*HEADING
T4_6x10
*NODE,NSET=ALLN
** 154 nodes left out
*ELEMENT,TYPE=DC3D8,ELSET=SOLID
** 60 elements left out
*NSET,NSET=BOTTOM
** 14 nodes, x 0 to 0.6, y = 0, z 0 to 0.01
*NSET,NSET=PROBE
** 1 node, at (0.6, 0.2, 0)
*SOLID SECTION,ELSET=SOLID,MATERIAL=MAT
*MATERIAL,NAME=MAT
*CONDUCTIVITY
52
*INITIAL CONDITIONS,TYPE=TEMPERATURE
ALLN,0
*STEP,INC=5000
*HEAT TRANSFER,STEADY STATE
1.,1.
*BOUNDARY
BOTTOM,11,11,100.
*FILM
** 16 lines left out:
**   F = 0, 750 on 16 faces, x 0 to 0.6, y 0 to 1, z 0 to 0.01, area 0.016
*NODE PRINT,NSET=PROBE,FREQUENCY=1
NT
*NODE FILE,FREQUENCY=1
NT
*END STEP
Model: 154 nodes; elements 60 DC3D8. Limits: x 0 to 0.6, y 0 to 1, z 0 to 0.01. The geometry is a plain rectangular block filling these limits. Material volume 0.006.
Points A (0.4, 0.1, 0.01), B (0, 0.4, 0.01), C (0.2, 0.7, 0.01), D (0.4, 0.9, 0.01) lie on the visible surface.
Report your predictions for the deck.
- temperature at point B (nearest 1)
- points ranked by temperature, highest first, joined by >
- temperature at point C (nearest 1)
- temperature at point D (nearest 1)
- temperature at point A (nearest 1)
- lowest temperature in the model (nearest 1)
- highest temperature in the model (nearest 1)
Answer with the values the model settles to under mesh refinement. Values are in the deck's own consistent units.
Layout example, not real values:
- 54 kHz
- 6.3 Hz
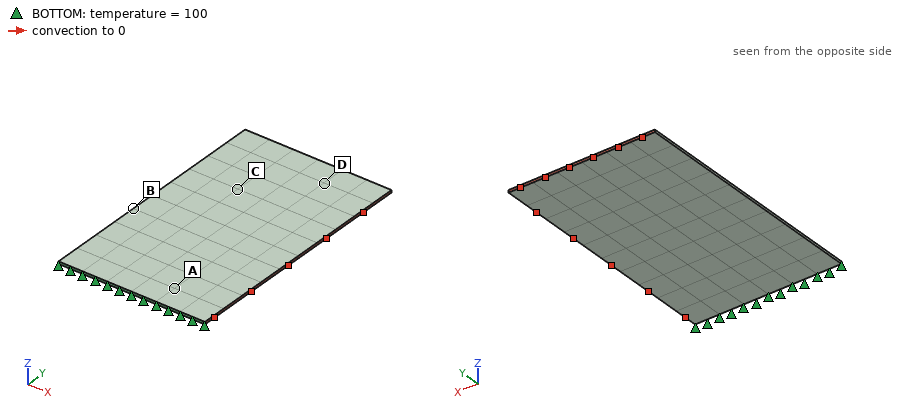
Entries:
- 45
- A > B > C > D
- 18
- 5
- 75
- 1
- 100
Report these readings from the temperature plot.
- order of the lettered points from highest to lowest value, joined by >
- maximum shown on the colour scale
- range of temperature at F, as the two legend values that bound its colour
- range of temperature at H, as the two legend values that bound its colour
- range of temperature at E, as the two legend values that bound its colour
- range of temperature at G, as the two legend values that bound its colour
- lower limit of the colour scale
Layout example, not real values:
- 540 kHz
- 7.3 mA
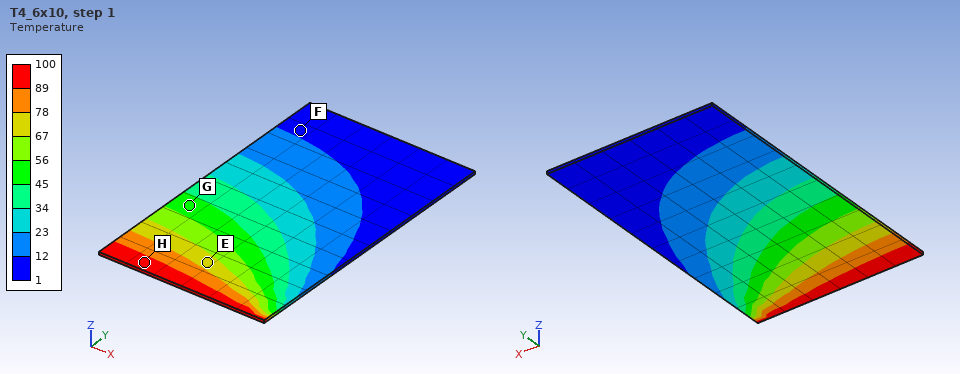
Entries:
- H > E > G > F
- 100
- 1 to 12
- 89 to 100
- 67 to 78
- 45 to 56
- 1
